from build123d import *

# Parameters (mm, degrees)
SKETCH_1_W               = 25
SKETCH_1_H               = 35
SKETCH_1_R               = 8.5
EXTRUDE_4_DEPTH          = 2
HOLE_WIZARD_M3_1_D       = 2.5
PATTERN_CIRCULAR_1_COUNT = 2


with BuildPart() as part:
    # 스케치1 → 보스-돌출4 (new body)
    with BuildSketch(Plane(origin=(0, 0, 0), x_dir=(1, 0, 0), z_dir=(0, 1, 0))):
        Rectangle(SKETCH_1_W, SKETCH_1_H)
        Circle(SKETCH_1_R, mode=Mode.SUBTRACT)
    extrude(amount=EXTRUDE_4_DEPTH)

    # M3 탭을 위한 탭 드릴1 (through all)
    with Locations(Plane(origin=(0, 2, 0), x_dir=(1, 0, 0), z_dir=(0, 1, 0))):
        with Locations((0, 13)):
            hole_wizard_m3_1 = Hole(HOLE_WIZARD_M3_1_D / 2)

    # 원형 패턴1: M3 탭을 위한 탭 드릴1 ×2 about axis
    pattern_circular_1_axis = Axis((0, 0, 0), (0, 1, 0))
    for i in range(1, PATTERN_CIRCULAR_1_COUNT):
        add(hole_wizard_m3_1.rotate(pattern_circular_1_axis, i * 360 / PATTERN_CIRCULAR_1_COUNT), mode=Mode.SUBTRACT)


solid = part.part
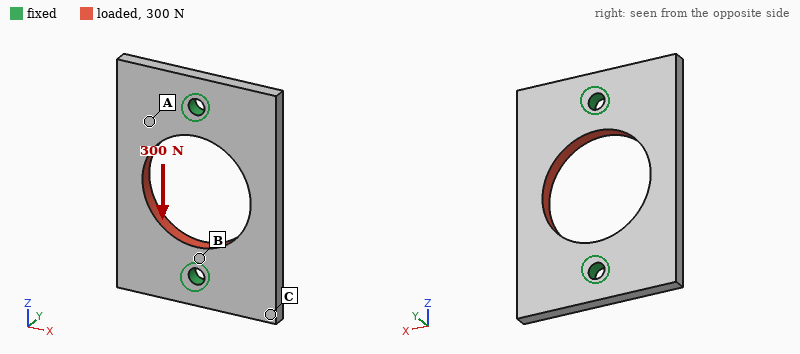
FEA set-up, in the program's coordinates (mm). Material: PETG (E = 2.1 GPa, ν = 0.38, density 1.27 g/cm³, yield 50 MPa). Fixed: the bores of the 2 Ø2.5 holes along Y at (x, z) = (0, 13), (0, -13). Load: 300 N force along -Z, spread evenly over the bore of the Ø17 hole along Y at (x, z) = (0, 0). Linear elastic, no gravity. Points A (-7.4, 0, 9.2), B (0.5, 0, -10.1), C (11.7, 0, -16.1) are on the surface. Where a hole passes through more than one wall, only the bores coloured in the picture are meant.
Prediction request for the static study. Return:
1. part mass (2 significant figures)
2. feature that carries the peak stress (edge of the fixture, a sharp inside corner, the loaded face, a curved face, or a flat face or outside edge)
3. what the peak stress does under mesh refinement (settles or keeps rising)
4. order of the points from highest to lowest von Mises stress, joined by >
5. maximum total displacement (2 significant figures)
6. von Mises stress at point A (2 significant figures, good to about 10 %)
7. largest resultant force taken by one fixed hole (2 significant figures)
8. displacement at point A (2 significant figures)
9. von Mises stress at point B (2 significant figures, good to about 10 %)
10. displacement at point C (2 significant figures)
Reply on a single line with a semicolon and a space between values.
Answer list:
1.6 g; edge of the fixture; keeps rising; B > A > C; 79 µm; 4.8 MPa; 150 N; 55 µm; 8.7 MPa; 68 µm
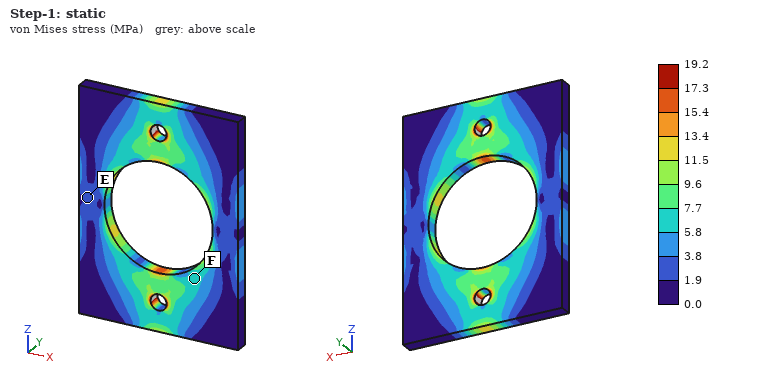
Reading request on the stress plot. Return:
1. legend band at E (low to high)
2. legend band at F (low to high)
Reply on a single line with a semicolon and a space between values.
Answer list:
1.9 to 3.8 MPa; 5.8 to 7.7 MPa
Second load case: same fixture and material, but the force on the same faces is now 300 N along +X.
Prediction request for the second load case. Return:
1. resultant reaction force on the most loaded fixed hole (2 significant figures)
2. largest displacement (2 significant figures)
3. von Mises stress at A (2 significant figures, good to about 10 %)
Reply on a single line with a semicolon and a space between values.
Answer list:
150 N; 90 µm; 5.0 MPa
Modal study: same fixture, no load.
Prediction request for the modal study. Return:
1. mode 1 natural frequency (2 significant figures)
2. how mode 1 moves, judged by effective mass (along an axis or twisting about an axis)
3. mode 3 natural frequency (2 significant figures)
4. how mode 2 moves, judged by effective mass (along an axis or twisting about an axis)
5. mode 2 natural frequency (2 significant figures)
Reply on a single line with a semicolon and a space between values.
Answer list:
1900 Hz; twisting about Z; 3100 Hz; along Y; 2000 Hz
